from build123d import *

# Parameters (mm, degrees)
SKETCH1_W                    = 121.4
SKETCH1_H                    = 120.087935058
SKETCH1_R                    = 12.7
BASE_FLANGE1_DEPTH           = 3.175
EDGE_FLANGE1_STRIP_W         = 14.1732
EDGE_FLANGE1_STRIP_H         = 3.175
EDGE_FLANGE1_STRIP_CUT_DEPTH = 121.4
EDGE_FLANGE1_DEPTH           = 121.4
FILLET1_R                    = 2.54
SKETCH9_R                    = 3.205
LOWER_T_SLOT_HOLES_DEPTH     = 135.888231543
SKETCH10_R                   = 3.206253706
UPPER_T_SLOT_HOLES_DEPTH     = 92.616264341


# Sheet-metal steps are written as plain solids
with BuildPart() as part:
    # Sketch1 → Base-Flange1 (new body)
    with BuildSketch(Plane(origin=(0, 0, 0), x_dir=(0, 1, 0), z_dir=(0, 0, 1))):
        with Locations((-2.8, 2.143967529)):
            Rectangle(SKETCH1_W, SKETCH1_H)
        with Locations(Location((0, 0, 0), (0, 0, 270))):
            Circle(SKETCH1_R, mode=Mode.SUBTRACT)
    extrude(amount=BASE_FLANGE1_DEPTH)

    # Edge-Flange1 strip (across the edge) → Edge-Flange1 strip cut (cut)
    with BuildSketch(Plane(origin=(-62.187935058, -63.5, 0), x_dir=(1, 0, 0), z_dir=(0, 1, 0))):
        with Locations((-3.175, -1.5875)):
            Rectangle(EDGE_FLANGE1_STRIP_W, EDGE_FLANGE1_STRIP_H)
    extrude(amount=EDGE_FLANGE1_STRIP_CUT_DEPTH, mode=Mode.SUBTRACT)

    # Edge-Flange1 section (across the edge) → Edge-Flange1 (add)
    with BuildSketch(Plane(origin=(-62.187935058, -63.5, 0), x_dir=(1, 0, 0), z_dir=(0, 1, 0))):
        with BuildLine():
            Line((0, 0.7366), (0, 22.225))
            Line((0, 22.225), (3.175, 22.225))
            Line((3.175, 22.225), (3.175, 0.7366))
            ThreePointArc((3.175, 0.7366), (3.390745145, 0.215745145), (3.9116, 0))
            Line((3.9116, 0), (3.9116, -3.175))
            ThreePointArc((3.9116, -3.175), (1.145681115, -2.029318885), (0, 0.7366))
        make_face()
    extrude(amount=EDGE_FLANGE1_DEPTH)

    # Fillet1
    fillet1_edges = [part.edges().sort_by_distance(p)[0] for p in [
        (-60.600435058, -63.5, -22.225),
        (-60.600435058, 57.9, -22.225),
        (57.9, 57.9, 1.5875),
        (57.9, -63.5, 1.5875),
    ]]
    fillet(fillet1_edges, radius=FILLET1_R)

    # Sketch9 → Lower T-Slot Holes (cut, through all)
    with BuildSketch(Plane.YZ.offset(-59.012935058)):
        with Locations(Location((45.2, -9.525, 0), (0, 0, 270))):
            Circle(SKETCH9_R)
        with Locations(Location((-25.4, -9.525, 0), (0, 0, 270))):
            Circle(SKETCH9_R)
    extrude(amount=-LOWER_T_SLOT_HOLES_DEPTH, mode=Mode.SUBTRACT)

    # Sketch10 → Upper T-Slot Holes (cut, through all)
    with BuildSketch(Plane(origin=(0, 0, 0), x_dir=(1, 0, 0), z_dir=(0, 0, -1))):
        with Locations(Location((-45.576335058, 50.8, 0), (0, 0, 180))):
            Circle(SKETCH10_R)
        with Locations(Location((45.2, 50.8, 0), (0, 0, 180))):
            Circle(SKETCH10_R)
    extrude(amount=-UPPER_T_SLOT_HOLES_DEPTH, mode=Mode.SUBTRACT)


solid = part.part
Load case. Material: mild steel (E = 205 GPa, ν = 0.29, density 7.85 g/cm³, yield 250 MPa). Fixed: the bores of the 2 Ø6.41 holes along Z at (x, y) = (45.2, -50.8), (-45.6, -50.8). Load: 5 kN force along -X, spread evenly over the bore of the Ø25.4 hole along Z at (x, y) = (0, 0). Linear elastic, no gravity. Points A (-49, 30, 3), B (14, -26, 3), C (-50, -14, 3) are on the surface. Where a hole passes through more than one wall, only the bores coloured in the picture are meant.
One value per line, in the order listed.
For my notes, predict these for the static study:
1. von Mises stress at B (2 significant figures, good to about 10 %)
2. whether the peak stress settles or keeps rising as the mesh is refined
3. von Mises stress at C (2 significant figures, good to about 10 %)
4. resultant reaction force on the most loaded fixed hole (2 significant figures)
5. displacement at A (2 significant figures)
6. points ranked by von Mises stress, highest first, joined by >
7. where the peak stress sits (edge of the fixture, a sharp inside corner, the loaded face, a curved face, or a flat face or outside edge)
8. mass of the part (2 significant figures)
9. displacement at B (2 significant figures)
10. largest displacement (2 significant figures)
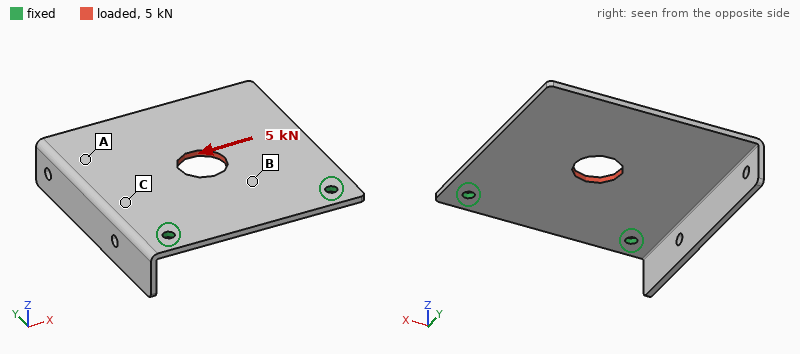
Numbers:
29 MPa
keeps rising
13 MPa
3.7 kN
21 µm
B > C > A
edge of the fixture
410 g
7.9 µm
26 µm
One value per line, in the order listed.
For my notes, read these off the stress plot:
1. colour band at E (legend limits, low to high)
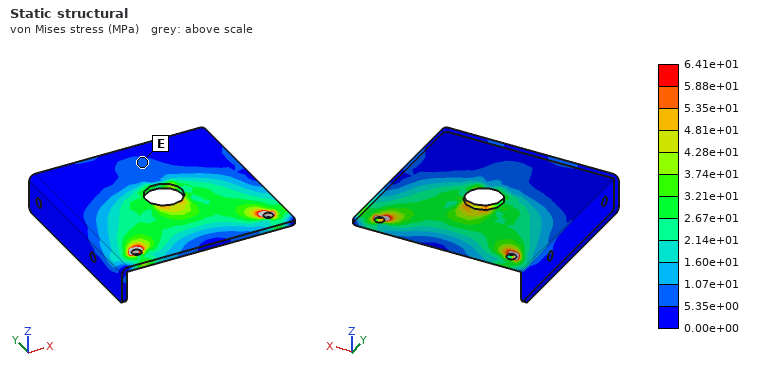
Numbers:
5.35e+00 to 1.07e+01 MPa
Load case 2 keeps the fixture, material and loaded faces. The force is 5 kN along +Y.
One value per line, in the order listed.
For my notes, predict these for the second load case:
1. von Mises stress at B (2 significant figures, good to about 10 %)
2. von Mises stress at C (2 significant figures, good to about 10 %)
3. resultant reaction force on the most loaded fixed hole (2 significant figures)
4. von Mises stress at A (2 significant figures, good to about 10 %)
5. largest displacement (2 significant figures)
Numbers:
16 MPa
11 MPa
2.6 kN
4.5 MPa
11 µm
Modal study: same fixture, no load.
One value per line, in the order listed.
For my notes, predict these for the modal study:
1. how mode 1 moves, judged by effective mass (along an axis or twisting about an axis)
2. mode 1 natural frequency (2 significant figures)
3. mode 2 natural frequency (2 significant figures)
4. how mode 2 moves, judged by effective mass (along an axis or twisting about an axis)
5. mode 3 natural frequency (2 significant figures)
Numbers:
along Z
260 Hz
480 Hz
twisting about Y
1100 Hz
